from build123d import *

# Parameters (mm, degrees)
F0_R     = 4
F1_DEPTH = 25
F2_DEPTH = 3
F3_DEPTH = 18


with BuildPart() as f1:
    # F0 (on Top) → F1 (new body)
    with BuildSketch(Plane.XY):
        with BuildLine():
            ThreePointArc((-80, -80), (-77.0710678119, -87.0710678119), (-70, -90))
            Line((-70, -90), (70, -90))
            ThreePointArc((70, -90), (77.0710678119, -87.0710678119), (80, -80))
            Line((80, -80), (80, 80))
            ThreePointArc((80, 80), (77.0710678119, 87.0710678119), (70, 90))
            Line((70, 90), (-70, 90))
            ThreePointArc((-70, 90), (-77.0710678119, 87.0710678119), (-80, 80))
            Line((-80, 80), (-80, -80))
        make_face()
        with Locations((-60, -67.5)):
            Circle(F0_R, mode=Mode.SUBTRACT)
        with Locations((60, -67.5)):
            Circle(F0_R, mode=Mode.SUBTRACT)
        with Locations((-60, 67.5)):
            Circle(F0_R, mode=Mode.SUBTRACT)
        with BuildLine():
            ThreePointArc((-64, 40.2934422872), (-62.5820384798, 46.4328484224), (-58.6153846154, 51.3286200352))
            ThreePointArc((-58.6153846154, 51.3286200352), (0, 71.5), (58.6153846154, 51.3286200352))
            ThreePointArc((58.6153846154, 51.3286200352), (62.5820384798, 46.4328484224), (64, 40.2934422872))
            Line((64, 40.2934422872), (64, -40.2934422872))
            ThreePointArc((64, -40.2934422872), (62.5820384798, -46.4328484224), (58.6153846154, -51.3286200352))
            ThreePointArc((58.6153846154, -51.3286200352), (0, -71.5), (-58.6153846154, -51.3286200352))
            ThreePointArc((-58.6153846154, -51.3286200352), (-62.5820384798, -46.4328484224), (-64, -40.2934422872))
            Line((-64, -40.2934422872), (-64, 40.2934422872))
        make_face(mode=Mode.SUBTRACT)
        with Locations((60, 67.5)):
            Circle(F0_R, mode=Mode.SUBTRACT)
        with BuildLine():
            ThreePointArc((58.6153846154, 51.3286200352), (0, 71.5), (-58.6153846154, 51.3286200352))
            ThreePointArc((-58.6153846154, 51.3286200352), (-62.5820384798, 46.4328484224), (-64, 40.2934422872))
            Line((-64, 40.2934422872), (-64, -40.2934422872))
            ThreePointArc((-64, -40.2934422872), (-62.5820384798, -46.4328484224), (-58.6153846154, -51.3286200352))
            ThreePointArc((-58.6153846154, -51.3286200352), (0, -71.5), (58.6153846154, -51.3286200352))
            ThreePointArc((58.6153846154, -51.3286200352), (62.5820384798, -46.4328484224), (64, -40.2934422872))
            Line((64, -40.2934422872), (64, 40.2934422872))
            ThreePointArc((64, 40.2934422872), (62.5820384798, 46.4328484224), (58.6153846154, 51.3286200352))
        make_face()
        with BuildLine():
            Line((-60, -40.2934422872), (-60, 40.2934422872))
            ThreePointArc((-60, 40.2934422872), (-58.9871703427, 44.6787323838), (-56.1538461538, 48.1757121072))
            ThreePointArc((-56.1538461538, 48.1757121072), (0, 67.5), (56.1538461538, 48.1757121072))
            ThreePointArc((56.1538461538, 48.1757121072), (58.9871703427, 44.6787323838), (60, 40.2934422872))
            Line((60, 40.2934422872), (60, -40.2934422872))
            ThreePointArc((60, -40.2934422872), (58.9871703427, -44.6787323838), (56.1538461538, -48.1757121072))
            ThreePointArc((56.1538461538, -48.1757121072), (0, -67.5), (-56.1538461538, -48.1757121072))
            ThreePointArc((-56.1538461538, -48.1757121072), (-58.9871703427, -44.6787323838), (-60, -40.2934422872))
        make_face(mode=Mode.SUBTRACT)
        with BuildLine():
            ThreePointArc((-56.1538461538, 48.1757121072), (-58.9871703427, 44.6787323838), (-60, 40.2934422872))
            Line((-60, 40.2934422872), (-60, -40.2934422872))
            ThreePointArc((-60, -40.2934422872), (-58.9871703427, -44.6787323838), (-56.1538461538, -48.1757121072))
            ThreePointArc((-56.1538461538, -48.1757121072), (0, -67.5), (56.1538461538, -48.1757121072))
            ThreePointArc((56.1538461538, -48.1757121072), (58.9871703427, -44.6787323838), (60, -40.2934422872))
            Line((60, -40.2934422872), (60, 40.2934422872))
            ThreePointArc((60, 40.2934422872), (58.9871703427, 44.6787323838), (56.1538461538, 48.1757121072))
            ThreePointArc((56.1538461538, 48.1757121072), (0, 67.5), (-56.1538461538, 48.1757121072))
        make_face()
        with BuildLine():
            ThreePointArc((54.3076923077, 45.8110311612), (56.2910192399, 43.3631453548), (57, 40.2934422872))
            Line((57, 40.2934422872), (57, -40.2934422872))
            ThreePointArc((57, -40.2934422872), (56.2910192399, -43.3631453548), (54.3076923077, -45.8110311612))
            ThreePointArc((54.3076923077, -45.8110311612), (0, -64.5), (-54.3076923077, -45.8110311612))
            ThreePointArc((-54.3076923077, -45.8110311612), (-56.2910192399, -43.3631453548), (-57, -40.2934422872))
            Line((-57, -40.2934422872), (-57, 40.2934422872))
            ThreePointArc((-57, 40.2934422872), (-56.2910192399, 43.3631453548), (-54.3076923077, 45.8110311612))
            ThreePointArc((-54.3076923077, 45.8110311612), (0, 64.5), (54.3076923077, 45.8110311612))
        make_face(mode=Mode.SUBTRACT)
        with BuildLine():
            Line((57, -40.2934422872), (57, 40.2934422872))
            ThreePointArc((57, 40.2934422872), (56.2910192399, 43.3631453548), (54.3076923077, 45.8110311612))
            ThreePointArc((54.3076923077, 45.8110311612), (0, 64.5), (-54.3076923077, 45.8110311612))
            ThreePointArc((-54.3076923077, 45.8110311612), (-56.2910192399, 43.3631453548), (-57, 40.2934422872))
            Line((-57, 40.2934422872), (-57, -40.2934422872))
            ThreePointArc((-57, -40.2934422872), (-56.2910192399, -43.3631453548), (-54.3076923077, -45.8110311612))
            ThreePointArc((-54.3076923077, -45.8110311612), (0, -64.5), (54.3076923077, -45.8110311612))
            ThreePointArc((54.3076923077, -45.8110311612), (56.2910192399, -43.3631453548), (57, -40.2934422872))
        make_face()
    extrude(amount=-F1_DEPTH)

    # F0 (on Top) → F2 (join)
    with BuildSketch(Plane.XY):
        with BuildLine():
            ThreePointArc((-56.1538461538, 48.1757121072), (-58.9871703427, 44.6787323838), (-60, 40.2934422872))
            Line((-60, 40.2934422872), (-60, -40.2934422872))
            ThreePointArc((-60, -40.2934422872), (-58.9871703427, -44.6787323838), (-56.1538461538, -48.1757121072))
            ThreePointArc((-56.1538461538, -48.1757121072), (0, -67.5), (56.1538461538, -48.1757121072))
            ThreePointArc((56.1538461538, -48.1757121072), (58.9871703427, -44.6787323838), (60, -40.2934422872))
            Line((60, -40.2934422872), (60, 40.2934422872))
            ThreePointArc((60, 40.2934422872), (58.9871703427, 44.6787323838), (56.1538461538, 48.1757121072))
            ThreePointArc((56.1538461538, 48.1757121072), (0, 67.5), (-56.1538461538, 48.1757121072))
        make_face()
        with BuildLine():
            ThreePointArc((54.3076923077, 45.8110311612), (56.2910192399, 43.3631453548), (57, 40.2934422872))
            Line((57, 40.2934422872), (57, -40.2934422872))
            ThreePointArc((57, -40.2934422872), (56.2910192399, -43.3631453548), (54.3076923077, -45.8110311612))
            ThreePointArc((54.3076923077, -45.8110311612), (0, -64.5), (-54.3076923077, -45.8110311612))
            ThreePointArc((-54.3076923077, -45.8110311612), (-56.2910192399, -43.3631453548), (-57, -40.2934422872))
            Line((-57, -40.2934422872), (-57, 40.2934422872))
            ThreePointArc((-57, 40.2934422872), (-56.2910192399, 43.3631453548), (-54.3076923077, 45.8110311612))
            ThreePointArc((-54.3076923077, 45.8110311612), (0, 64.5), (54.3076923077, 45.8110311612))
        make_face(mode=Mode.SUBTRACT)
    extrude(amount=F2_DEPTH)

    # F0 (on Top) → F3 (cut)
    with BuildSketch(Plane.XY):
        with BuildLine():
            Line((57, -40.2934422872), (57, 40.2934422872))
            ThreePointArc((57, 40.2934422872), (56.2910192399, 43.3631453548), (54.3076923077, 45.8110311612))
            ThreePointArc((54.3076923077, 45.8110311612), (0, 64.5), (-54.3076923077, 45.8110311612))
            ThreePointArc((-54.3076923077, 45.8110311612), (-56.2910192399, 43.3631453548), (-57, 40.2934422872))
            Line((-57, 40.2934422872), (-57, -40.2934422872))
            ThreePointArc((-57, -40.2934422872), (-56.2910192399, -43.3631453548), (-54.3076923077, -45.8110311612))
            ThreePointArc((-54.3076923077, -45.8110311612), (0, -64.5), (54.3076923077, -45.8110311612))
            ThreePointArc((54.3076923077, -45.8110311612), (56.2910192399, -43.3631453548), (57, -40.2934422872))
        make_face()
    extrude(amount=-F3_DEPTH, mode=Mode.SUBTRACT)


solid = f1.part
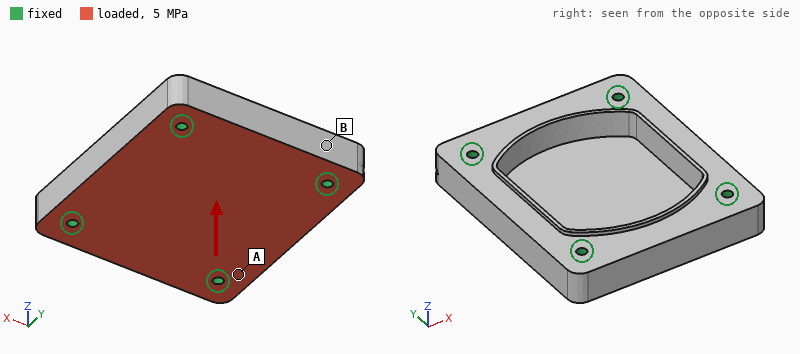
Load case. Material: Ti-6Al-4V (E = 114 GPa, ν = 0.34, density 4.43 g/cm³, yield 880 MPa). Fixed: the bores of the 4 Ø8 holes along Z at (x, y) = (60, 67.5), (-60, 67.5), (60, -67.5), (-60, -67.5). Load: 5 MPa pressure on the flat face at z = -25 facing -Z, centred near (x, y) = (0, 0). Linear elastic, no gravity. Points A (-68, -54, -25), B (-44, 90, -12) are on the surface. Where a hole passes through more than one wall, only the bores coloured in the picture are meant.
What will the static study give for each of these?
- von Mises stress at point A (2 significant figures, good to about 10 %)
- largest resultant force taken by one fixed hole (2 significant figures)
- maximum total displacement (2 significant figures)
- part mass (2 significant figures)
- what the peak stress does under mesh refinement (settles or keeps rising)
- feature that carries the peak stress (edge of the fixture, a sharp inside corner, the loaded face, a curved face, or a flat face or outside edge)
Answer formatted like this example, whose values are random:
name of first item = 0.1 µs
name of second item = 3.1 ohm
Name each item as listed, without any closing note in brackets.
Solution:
von Mises stress at point A = 60 MPa
largest resultant force taken by one fixed hole = 37 kN
maximum total displacement = 0.57 mm
part mass = 2.1 kg
what the peak stress does under mesh refinement = keeps rising
feature that carries the peak stress = edge of the fixture
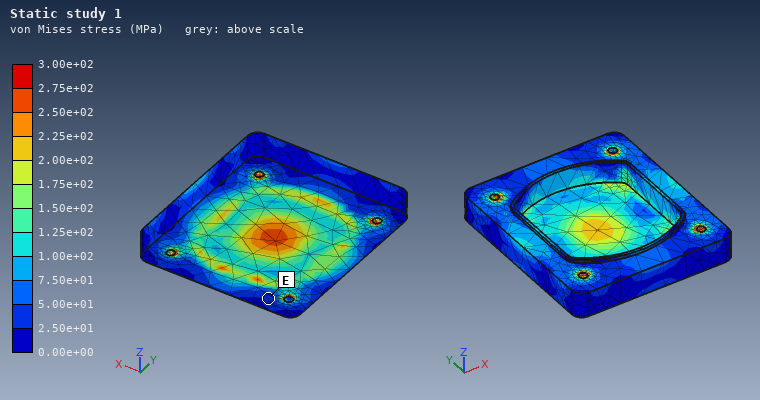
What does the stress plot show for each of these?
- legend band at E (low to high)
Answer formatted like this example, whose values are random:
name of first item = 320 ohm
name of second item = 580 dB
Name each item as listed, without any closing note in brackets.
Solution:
legend band at E = 2.50e+01 to 5.00e+01 MPa
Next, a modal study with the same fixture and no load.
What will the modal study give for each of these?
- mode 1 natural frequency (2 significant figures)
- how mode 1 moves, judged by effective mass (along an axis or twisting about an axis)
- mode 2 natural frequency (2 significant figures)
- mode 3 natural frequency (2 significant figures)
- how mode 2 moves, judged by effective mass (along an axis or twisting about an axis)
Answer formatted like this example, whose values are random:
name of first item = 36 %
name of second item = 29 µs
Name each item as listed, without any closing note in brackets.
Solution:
mode 1 natural frequency = 3400 Hz
how mode 1 moves, judged by effective mass = along Z
mode 2 natural frequency = 5500 Hz
mode 3 natural frequency = 6000 Hz
how mode 2 moves, judged by effective mass = twisting about Y
